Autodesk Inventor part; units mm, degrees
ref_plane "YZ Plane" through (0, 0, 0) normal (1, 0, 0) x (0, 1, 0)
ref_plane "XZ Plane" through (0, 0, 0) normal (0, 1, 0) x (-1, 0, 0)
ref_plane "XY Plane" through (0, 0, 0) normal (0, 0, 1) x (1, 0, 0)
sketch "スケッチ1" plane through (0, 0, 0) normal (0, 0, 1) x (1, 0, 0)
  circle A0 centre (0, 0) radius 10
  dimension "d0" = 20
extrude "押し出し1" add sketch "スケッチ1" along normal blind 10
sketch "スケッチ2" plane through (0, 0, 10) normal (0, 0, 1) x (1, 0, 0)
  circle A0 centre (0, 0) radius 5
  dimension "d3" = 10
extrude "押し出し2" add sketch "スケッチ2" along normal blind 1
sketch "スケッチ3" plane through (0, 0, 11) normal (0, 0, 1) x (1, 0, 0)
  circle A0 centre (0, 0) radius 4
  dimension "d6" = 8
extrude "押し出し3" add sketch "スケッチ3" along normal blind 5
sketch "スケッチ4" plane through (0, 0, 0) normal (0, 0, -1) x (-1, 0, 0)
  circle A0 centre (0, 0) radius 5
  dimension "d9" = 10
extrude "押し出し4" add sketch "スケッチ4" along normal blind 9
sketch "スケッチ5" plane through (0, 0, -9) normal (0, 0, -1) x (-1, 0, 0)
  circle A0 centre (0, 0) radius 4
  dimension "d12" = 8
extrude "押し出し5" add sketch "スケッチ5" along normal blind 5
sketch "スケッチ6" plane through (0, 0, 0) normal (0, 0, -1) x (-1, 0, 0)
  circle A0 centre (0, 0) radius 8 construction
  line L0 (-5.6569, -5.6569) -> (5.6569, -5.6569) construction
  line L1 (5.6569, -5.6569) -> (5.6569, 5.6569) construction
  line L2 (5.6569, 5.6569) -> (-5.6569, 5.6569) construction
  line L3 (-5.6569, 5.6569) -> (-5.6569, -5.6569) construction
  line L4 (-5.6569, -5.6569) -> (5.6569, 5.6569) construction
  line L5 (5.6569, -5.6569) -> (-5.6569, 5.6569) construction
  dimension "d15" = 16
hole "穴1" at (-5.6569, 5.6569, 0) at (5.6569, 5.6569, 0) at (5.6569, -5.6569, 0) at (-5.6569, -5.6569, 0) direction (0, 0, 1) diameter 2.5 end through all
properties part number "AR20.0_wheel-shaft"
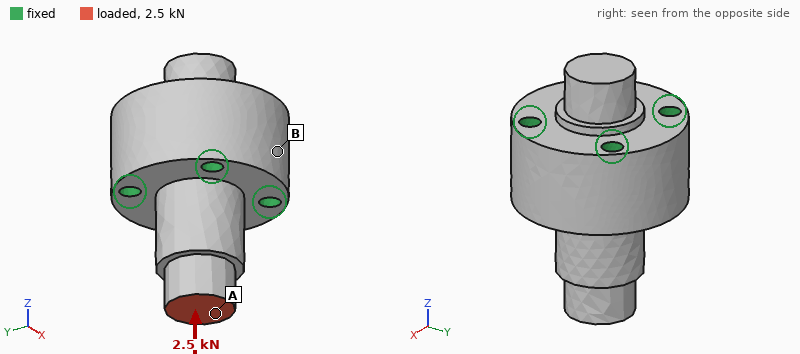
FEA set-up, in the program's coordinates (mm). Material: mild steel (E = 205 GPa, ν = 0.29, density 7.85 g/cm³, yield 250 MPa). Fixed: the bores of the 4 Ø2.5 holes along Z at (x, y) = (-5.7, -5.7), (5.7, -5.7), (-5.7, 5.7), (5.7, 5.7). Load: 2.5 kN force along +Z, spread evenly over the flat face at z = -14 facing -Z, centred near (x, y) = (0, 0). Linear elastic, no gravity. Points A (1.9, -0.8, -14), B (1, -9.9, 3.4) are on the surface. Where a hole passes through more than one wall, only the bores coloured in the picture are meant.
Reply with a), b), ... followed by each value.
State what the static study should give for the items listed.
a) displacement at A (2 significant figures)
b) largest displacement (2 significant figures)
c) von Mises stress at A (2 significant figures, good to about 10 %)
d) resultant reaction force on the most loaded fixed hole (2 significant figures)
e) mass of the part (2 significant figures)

a) 3.4 µm
b) 3.4 µm
c) 51 MPa
d) 660 N
e) 33 g
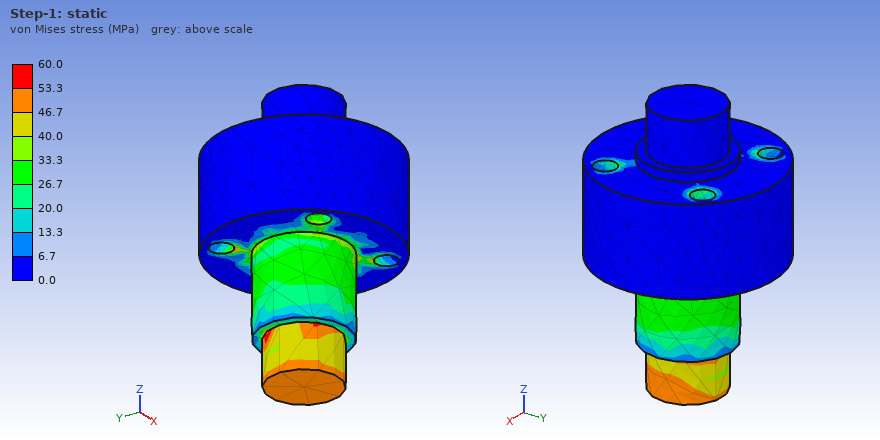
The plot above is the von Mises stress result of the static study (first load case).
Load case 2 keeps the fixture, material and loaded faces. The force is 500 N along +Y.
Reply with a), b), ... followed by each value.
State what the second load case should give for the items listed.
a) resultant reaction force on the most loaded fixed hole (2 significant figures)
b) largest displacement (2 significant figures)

a) 380 N
b) 9.5 µm
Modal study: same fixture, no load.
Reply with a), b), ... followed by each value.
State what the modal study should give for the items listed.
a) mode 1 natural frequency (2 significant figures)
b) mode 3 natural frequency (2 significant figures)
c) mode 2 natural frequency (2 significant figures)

a) 27 kHz
b) 62 kHz
c) 27 kHz
